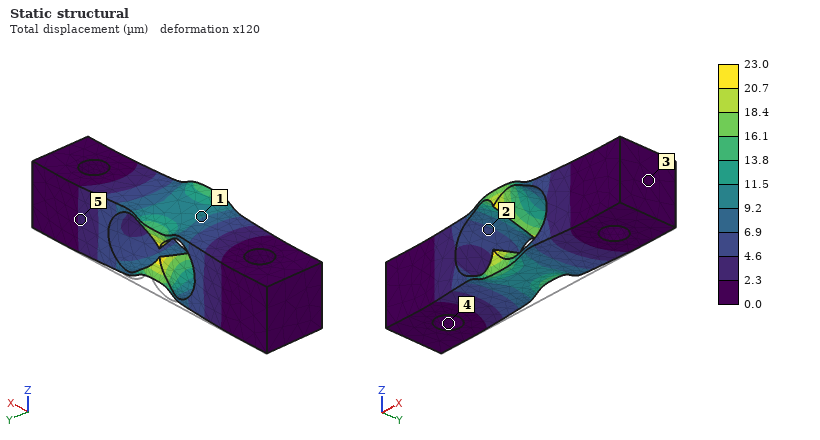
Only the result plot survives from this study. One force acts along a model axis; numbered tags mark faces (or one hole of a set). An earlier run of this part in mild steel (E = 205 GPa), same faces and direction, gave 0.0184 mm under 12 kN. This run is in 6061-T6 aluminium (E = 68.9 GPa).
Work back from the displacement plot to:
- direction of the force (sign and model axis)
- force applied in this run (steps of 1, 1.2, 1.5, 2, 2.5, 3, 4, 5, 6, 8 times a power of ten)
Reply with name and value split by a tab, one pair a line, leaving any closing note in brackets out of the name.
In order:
direction of the force	-Y
force applied in this run	5 kN
